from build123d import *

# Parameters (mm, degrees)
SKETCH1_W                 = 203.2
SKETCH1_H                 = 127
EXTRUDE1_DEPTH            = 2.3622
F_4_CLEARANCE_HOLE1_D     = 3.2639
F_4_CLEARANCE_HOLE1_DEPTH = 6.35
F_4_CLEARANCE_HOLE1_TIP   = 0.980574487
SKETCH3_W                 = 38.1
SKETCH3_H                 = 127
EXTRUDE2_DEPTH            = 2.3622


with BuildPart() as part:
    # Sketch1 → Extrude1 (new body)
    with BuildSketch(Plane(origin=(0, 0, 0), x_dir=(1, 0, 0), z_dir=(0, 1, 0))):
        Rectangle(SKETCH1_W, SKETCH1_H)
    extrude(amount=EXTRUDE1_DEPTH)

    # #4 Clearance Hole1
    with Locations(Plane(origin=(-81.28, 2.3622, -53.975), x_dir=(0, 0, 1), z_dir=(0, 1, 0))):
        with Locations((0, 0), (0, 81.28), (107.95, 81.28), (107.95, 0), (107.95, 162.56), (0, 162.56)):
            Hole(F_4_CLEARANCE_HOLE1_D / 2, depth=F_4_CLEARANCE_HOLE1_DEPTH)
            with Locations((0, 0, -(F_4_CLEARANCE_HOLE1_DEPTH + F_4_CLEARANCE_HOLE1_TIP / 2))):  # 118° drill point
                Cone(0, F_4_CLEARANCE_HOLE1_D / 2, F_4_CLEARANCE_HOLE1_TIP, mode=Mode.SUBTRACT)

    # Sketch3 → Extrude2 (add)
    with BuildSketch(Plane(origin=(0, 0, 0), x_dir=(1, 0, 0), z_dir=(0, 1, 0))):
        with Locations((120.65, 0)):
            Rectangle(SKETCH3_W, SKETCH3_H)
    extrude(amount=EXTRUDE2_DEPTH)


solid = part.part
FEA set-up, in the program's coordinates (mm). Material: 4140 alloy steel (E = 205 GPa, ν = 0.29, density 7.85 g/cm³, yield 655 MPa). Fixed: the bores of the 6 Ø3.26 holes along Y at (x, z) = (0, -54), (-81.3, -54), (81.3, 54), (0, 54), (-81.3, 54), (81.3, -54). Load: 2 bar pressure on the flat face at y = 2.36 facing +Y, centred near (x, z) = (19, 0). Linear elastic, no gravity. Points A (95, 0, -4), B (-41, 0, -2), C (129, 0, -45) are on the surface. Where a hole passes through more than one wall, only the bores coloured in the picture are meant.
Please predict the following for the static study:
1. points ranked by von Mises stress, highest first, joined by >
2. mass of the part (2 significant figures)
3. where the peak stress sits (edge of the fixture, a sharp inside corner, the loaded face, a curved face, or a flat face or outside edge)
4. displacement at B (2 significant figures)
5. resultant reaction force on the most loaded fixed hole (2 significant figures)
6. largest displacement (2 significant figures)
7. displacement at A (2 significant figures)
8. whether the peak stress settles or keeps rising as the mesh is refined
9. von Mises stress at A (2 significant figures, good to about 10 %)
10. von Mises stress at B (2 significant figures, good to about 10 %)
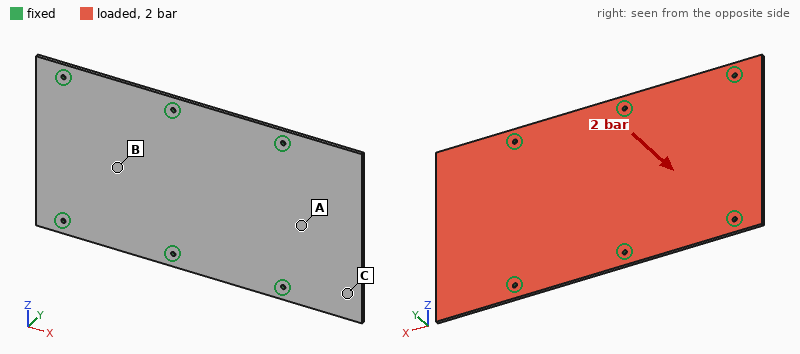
A > B > C
570 g
edge of the fixture
0.56 mm
1.3 kN
2.4 mm
0.95 mm
keeps rising
230 MPa
110 MPa
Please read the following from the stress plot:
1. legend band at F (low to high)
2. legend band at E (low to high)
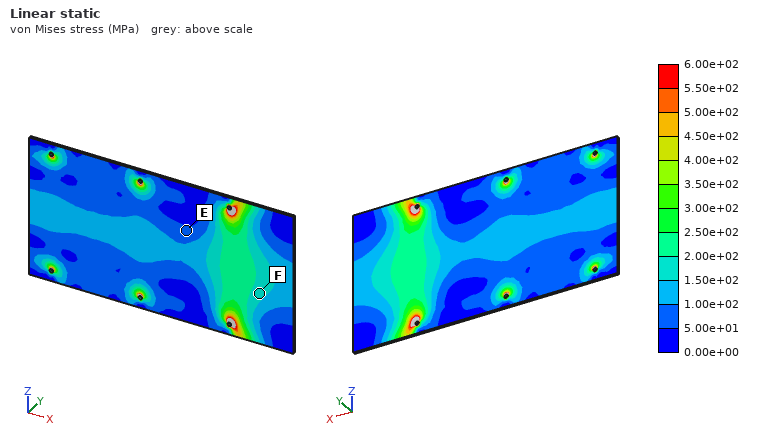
1.50e+02 to 2.00e+02 MPa
5.00e+01 to 1.00e+02 MPa
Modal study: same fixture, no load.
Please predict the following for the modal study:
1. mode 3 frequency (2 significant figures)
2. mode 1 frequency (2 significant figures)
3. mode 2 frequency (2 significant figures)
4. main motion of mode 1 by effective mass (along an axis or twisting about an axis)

810 Hz
420 Hz
810 Hz
along Y
